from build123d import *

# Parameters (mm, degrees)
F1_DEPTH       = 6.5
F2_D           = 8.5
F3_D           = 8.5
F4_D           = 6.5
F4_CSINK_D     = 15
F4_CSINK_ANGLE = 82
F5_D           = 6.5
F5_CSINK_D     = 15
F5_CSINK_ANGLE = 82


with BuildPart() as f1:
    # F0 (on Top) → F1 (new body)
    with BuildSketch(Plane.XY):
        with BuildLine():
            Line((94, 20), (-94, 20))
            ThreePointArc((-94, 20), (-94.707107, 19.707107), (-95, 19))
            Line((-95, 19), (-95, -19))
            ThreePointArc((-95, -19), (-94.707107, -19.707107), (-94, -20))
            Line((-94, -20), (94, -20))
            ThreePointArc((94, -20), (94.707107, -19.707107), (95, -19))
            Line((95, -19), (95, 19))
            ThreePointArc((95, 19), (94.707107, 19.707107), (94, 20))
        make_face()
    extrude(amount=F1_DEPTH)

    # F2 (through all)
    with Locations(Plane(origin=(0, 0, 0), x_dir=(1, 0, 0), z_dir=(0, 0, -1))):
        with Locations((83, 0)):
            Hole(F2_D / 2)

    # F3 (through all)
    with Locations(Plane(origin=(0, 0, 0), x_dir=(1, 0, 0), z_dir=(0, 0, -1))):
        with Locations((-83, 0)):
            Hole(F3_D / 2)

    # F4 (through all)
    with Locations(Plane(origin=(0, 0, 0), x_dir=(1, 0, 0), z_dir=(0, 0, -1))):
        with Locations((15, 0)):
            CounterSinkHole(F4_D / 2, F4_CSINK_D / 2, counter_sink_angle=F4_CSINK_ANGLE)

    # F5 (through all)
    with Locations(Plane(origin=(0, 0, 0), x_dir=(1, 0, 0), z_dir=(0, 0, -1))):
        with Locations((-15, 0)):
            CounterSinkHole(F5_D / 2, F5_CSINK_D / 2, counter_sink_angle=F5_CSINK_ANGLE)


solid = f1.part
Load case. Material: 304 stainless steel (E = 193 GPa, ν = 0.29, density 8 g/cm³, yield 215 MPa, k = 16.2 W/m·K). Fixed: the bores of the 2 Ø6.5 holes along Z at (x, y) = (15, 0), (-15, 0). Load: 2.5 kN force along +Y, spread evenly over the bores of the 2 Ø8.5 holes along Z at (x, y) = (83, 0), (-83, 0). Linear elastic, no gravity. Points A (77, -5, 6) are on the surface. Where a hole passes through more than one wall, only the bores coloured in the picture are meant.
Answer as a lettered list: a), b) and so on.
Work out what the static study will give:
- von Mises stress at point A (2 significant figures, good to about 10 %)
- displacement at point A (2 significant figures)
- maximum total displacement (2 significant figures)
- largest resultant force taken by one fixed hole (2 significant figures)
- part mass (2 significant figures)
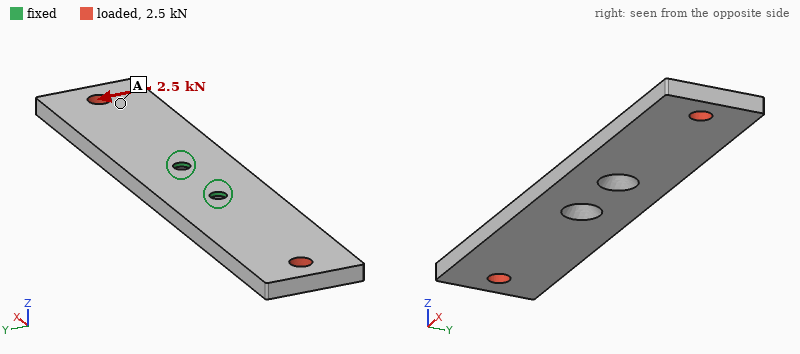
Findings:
a) 9.5 MPa
b) 33 µm
c) 51 µm
d) 1.3 kN
e) 380 g
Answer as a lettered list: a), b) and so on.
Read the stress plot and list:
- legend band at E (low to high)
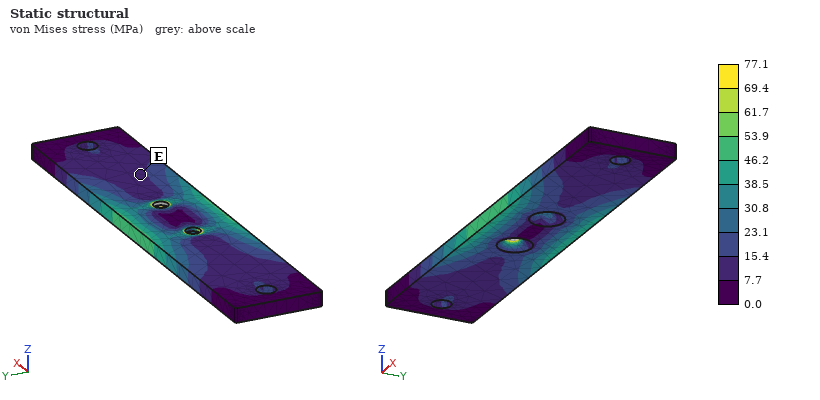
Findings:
a) 7.7 to 15.4 MPa
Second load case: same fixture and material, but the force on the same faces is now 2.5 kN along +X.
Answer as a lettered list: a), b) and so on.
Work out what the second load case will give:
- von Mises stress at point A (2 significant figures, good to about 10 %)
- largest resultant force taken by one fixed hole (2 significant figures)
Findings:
a) 8.6 MPa
b) 1.3 kN
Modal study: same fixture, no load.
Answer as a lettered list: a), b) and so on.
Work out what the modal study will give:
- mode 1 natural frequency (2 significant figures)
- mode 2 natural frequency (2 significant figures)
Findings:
a) 700 Hz
b) 710 Hz
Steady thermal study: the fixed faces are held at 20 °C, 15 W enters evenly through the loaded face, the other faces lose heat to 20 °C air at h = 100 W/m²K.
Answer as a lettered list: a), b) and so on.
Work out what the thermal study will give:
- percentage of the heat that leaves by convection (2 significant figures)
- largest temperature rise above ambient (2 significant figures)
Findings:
a) 97 %
b) 33 K
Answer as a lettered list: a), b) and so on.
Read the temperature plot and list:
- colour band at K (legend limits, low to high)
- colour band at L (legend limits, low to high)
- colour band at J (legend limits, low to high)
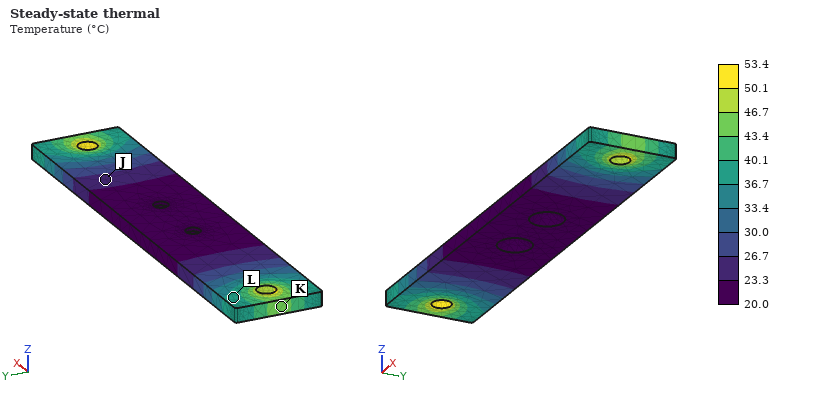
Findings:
a) 43.4 to 46.7 °C
b) 36.7 to 40.1 °C
c) 23.3 to 26.7 °C
